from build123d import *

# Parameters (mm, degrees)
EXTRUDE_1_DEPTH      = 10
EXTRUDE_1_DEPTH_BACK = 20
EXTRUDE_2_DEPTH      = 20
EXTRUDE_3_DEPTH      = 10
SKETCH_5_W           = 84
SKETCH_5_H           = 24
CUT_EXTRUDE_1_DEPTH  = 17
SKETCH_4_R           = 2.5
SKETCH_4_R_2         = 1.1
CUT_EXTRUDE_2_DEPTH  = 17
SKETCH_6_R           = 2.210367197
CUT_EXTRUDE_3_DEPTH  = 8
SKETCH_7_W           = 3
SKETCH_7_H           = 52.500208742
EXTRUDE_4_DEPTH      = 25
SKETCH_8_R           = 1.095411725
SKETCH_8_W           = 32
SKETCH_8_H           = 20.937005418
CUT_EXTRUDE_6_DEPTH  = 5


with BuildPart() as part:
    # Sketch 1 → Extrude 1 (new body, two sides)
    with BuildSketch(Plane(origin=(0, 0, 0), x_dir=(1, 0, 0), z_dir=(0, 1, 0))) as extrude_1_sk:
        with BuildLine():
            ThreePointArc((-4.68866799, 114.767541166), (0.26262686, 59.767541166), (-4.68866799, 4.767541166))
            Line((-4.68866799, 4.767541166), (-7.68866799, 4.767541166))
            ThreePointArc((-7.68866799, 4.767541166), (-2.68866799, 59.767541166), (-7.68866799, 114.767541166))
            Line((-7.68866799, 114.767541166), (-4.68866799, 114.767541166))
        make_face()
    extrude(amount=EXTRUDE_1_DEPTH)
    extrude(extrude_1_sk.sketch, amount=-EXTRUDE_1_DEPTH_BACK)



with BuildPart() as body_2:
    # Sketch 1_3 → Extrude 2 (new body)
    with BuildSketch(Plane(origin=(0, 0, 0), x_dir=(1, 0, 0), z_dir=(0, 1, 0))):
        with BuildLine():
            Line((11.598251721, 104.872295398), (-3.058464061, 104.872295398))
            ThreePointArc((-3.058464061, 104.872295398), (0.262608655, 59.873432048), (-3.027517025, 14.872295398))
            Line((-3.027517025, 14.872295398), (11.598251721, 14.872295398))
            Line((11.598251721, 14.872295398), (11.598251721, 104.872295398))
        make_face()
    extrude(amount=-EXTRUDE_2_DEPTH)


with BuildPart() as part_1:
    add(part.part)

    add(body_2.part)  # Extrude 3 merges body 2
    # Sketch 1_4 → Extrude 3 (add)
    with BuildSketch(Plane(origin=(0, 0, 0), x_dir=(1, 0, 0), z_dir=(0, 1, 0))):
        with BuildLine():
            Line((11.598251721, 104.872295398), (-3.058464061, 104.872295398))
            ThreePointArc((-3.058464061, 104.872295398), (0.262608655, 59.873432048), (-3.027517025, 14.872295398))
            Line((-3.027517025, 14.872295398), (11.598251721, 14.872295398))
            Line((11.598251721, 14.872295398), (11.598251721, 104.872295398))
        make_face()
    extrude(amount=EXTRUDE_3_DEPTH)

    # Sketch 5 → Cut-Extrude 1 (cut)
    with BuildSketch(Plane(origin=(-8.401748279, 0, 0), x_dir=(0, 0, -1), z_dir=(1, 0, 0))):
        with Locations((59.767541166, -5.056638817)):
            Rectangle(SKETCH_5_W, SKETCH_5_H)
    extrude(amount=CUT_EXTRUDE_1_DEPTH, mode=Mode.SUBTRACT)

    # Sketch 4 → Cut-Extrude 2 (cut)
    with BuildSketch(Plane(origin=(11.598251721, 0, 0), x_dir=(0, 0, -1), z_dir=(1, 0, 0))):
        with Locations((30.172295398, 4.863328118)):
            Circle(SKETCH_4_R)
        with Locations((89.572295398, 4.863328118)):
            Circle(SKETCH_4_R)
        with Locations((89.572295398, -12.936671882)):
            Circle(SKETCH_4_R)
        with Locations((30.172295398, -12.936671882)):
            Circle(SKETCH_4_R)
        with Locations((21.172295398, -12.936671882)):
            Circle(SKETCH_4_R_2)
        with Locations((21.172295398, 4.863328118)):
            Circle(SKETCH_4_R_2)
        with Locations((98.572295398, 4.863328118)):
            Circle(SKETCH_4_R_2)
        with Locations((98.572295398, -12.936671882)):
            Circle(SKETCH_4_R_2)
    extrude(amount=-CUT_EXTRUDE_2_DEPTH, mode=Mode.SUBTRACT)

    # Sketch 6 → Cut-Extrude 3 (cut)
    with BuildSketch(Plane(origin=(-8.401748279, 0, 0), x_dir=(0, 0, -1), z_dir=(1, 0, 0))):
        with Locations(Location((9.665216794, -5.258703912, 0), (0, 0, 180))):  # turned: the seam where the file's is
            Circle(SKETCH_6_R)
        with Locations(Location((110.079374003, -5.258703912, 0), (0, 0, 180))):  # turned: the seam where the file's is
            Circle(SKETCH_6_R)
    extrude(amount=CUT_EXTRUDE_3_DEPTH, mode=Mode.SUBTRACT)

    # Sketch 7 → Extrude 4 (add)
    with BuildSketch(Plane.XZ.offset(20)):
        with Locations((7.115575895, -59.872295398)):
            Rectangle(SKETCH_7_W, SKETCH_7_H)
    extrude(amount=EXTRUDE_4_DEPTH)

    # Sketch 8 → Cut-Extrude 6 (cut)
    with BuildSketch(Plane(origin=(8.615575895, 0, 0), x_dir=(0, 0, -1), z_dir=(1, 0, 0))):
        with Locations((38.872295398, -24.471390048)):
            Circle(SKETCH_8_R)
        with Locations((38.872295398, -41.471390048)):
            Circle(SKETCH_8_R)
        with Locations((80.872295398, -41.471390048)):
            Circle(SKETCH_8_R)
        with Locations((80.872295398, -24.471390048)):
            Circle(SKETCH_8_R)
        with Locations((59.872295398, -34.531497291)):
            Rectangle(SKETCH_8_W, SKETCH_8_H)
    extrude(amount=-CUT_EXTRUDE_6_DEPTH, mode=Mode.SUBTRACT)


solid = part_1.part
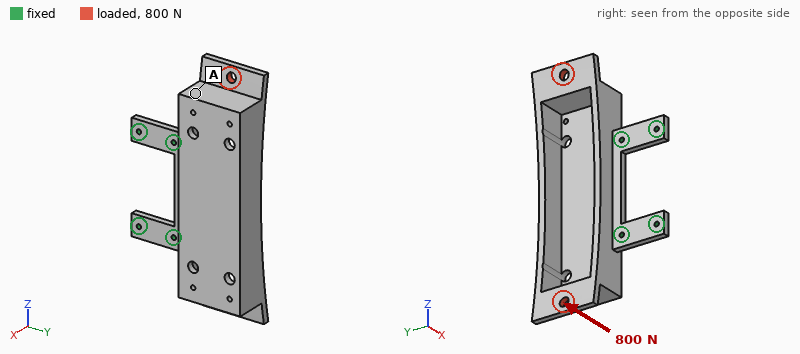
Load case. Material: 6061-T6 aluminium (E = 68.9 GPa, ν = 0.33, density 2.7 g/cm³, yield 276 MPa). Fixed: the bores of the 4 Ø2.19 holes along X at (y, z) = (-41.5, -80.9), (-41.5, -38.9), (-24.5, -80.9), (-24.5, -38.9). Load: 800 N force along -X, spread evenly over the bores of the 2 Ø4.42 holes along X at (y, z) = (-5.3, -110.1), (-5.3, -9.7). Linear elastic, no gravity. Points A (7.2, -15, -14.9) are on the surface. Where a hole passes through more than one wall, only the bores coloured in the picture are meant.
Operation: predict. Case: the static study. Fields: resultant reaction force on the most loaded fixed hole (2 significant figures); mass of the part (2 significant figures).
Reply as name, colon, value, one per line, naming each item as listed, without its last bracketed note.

resultant reaction force on the most loaded fixed hole: 490 N
mass of the part: 54 g
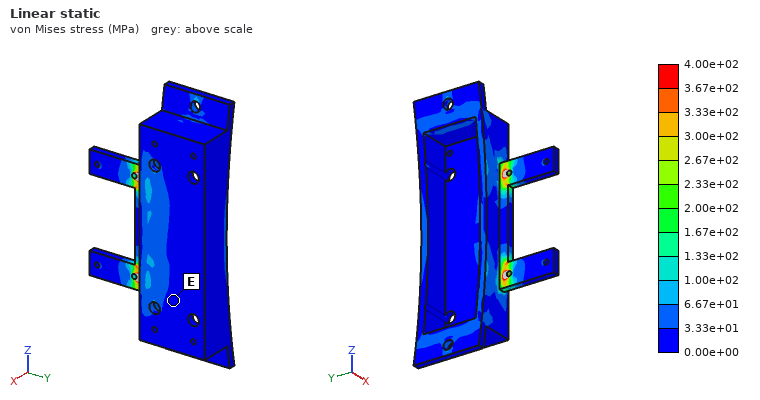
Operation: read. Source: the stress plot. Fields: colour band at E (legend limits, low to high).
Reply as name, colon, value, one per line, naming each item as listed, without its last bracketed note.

colour band at E: 0.00e+00 to 3.33e+01 MPa
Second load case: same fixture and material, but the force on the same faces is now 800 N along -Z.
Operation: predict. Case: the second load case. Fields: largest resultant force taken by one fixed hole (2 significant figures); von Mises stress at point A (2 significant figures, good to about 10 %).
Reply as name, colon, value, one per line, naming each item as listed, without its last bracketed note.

largest resultant force taken by one fixed hole: 570 N
von Mises stress at point A: 17 MPa
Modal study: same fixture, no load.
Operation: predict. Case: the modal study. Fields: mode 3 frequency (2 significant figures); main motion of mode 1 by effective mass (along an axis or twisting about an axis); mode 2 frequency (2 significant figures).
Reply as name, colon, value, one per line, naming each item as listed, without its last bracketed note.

mode 3 frequency: 4200 Hz
main motion of mode 1 by effective mass: along X
mode 2 frequency: 1400 Hz
